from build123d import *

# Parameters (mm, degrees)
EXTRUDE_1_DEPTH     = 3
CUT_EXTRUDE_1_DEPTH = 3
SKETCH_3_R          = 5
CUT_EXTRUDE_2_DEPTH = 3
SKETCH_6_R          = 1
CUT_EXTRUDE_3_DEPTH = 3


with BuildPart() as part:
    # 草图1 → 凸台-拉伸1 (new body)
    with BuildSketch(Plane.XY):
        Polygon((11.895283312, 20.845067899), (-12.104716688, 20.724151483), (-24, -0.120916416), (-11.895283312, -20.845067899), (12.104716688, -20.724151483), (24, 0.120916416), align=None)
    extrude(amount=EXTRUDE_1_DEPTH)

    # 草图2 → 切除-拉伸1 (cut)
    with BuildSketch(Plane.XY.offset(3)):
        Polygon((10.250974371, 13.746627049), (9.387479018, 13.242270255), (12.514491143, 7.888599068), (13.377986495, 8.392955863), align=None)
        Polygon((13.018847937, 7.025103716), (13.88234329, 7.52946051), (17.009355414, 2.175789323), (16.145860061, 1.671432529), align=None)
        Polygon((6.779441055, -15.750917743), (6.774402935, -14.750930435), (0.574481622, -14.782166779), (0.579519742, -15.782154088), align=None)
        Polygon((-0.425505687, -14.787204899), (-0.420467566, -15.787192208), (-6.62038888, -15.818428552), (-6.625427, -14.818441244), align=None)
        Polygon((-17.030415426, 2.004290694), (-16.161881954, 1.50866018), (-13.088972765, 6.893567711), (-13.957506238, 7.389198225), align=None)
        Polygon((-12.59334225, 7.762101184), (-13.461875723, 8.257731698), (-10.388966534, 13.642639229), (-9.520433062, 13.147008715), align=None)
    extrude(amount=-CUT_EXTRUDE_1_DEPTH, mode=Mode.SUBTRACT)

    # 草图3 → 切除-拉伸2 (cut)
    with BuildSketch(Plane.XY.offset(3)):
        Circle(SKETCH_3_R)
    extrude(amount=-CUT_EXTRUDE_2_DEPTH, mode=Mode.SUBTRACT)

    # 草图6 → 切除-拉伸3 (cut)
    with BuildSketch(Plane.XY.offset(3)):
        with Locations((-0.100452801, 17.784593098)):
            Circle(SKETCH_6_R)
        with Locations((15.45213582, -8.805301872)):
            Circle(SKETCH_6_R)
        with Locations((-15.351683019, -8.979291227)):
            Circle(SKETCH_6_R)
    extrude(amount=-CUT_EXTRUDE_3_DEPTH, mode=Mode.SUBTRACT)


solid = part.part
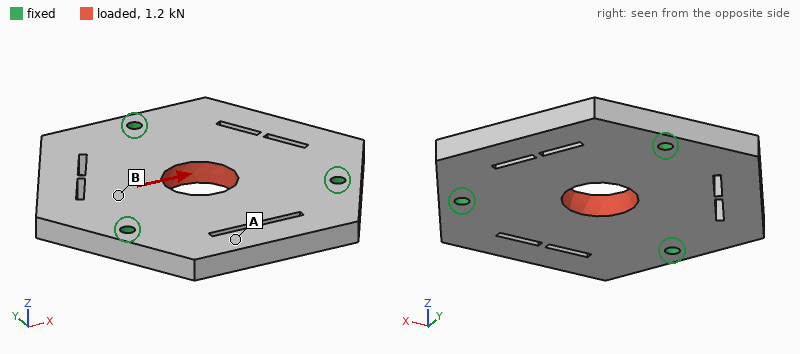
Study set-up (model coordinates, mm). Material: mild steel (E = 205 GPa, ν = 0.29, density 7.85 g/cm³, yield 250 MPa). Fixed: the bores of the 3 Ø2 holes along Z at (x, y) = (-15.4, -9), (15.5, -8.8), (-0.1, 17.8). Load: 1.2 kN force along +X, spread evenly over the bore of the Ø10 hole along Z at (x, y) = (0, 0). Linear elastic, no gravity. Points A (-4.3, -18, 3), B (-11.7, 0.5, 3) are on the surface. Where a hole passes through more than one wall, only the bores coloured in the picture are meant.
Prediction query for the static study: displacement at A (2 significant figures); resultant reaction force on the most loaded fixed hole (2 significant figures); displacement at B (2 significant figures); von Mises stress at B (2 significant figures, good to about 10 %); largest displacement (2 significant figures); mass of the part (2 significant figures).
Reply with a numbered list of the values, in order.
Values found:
1. 0.36 µm
2. 410 N
3. 1.0 µm
4. 11 MPa
5. 1.6 µm
6. 32 g
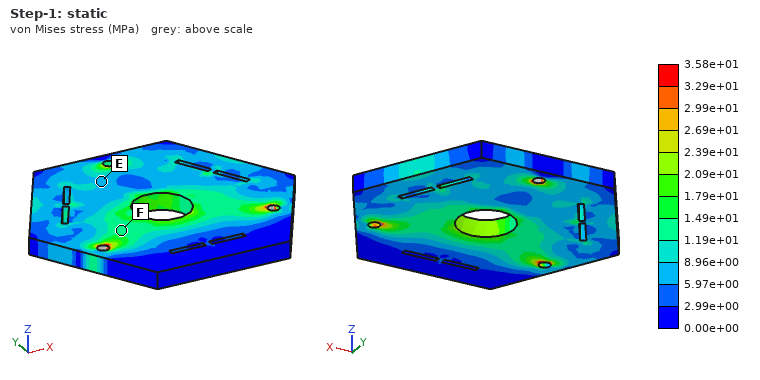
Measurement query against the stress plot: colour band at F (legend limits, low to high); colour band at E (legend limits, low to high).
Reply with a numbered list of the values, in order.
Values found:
1. 1.19e+01 to 1.49e+01 MPa
2. 5.97e+00 to 8.96e+00 MPa
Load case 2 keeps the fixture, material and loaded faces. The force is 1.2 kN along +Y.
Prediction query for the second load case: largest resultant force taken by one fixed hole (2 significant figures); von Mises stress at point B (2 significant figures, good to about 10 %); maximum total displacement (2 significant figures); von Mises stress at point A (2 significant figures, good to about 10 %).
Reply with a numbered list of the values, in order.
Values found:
1. 410 N
2. 6.7 MPa
3. 1.7 µm
4. 7.5 MPa
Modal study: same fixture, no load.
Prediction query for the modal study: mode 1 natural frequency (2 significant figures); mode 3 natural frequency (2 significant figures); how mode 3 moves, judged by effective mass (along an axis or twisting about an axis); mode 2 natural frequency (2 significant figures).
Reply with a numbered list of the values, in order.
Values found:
1. 9900 Hz
2. 12 kHz
3. along Z
4. 9900 Hz
